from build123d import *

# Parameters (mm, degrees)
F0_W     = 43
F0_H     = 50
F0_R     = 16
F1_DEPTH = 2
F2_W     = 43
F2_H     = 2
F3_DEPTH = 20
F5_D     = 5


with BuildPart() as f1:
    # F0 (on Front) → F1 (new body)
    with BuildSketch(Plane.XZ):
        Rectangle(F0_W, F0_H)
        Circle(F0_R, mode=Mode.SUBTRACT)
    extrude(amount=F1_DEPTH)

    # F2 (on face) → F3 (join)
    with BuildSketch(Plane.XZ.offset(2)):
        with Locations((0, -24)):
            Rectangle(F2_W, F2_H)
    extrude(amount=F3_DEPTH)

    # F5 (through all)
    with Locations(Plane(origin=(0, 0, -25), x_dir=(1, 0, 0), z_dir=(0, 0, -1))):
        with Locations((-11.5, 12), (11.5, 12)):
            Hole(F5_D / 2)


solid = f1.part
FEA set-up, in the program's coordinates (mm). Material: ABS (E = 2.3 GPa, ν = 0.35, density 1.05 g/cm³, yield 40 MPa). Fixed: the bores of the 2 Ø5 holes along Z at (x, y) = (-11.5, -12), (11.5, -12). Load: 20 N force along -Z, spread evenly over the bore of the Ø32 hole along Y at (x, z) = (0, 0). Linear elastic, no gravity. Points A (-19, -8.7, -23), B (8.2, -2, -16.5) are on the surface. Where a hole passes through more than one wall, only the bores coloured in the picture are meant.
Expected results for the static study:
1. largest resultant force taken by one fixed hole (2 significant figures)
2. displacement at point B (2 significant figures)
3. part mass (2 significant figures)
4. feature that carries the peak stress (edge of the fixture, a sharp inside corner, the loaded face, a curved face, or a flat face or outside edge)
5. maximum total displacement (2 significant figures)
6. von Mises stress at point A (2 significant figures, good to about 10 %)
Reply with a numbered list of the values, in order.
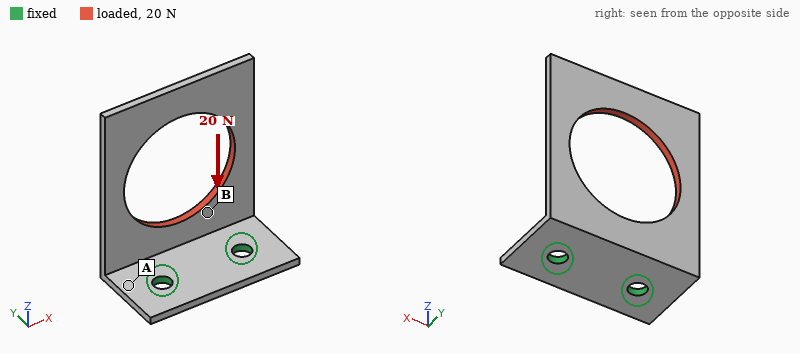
1. 10 N
2. 0.14 mm
3. 4.5 g
4. a flat face or outside edge
5. 0.72 mm
6. 3.4 MPa
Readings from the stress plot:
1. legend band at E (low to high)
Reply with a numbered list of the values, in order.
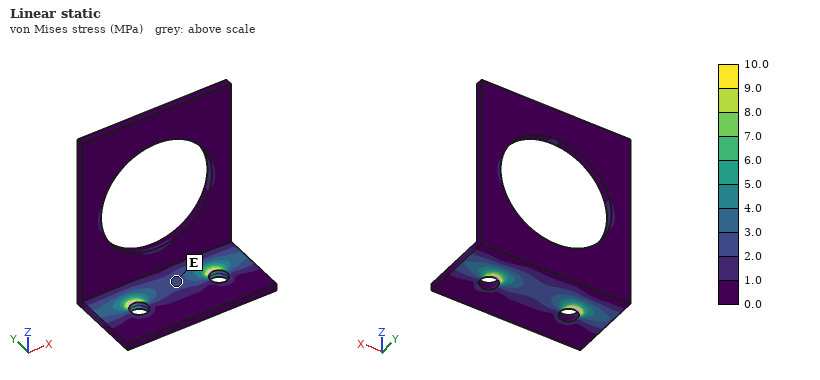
1. 2.0 to 3.0 MPa
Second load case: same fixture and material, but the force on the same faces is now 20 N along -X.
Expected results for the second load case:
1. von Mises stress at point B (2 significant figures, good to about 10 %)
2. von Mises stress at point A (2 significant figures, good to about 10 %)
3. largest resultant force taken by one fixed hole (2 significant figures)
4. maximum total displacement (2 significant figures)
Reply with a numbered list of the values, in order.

1. 2.6 MPa
2. 5.2 MPa
3. 22 N
4. 0.71 mm
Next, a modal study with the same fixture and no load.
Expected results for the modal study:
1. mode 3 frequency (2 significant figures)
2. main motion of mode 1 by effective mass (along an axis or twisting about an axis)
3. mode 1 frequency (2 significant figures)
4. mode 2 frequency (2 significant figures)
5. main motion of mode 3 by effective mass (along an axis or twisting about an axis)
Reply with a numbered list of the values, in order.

1. 620 Hz
2. along Y
3. 140 Hz
4. 380 Hz
5. along X
